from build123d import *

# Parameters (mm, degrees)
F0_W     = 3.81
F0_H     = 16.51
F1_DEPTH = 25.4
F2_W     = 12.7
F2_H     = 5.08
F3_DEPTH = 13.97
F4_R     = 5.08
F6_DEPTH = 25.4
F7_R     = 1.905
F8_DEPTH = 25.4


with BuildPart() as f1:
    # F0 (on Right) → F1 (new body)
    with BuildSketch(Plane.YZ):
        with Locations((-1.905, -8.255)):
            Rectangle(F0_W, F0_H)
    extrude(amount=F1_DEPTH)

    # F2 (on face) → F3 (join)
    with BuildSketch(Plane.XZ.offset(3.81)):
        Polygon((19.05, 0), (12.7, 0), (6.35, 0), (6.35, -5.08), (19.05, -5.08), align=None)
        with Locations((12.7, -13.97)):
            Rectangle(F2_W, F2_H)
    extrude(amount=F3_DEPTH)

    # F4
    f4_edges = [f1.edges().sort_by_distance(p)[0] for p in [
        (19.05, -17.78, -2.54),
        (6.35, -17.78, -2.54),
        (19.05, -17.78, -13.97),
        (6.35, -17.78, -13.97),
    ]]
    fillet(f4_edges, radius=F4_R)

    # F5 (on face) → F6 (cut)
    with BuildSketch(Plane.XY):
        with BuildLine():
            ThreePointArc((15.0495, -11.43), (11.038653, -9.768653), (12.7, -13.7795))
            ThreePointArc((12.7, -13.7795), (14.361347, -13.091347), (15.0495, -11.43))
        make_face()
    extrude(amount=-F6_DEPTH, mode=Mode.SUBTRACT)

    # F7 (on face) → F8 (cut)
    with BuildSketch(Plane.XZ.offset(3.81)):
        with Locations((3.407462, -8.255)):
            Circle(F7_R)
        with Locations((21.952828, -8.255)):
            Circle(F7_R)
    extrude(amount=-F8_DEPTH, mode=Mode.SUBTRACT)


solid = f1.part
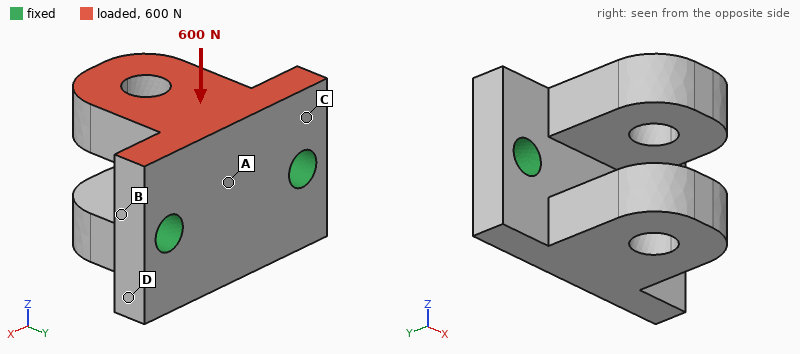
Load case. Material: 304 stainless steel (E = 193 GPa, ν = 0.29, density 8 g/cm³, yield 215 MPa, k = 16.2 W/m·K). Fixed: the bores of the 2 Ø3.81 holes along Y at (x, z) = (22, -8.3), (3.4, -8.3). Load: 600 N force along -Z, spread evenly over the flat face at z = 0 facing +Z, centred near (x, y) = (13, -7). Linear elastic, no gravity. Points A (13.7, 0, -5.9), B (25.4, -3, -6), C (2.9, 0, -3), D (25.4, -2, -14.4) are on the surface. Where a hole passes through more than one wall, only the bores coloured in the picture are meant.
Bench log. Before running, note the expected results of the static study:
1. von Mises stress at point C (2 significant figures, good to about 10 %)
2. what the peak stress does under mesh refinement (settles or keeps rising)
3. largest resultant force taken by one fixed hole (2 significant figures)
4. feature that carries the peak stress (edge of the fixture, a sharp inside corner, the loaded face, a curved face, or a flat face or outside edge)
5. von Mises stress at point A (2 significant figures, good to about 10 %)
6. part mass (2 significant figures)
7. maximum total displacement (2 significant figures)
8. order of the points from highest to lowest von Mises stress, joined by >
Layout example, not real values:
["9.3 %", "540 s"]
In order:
["27 MPa", "keeps rising", "310 N", "edge of the fixture", "37 MPa", "24 g", "20 µm", "A > C > B > D"]
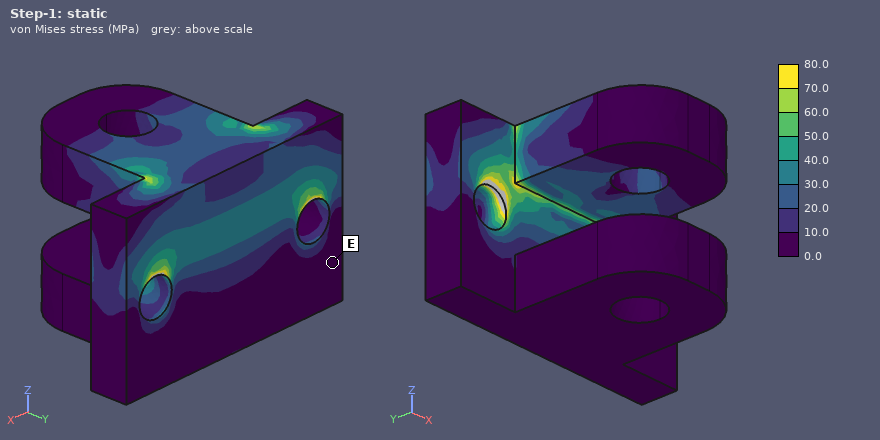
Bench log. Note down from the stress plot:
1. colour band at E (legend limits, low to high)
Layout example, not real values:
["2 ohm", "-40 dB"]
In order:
["0.0 to 10.0 MPa"]
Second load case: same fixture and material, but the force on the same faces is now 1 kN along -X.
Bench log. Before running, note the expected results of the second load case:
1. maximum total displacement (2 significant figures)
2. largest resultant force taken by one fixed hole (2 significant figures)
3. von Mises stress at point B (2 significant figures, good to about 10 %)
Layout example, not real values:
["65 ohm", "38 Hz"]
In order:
["7.9 µm", "710 N", "10 MPa"]
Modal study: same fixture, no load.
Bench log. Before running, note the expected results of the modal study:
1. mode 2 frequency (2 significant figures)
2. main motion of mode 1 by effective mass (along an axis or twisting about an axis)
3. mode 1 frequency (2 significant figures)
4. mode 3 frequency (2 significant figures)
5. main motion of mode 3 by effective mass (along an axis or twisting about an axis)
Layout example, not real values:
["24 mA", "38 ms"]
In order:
["11 kHz", "along Z", "9900 Hz", "21 kHz", "along X"]
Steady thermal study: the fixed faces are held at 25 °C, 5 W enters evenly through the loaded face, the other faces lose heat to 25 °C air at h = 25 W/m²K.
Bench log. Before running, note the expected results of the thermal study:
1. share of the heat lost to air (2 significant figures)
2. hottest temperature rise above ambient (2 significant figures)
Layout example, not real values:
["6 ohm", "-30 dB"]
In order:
["11 %", "45 K"]
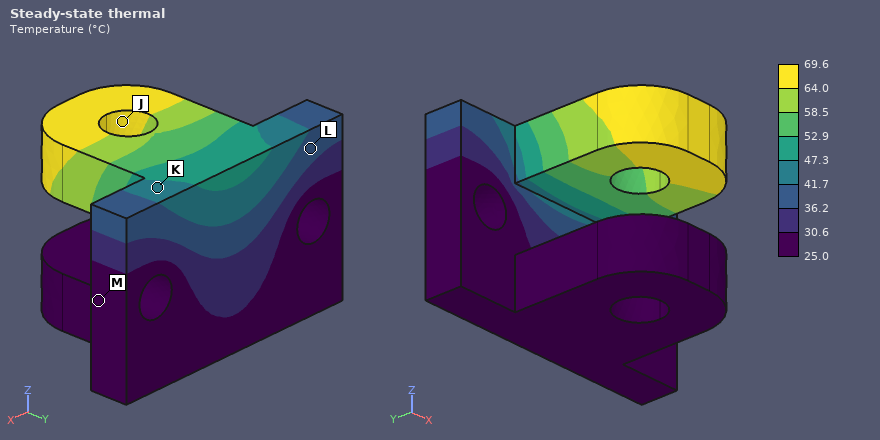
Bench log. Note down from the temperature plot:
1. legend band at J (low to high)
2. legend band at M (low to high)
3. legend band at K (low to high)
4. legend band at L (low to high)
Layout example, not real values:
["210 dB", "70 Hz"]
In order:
["64.0 to 69.6 °C", "25.0 to 30.6 °C", "41.7 to 47.3 °C", "36.2 to 41.7 °C"]
